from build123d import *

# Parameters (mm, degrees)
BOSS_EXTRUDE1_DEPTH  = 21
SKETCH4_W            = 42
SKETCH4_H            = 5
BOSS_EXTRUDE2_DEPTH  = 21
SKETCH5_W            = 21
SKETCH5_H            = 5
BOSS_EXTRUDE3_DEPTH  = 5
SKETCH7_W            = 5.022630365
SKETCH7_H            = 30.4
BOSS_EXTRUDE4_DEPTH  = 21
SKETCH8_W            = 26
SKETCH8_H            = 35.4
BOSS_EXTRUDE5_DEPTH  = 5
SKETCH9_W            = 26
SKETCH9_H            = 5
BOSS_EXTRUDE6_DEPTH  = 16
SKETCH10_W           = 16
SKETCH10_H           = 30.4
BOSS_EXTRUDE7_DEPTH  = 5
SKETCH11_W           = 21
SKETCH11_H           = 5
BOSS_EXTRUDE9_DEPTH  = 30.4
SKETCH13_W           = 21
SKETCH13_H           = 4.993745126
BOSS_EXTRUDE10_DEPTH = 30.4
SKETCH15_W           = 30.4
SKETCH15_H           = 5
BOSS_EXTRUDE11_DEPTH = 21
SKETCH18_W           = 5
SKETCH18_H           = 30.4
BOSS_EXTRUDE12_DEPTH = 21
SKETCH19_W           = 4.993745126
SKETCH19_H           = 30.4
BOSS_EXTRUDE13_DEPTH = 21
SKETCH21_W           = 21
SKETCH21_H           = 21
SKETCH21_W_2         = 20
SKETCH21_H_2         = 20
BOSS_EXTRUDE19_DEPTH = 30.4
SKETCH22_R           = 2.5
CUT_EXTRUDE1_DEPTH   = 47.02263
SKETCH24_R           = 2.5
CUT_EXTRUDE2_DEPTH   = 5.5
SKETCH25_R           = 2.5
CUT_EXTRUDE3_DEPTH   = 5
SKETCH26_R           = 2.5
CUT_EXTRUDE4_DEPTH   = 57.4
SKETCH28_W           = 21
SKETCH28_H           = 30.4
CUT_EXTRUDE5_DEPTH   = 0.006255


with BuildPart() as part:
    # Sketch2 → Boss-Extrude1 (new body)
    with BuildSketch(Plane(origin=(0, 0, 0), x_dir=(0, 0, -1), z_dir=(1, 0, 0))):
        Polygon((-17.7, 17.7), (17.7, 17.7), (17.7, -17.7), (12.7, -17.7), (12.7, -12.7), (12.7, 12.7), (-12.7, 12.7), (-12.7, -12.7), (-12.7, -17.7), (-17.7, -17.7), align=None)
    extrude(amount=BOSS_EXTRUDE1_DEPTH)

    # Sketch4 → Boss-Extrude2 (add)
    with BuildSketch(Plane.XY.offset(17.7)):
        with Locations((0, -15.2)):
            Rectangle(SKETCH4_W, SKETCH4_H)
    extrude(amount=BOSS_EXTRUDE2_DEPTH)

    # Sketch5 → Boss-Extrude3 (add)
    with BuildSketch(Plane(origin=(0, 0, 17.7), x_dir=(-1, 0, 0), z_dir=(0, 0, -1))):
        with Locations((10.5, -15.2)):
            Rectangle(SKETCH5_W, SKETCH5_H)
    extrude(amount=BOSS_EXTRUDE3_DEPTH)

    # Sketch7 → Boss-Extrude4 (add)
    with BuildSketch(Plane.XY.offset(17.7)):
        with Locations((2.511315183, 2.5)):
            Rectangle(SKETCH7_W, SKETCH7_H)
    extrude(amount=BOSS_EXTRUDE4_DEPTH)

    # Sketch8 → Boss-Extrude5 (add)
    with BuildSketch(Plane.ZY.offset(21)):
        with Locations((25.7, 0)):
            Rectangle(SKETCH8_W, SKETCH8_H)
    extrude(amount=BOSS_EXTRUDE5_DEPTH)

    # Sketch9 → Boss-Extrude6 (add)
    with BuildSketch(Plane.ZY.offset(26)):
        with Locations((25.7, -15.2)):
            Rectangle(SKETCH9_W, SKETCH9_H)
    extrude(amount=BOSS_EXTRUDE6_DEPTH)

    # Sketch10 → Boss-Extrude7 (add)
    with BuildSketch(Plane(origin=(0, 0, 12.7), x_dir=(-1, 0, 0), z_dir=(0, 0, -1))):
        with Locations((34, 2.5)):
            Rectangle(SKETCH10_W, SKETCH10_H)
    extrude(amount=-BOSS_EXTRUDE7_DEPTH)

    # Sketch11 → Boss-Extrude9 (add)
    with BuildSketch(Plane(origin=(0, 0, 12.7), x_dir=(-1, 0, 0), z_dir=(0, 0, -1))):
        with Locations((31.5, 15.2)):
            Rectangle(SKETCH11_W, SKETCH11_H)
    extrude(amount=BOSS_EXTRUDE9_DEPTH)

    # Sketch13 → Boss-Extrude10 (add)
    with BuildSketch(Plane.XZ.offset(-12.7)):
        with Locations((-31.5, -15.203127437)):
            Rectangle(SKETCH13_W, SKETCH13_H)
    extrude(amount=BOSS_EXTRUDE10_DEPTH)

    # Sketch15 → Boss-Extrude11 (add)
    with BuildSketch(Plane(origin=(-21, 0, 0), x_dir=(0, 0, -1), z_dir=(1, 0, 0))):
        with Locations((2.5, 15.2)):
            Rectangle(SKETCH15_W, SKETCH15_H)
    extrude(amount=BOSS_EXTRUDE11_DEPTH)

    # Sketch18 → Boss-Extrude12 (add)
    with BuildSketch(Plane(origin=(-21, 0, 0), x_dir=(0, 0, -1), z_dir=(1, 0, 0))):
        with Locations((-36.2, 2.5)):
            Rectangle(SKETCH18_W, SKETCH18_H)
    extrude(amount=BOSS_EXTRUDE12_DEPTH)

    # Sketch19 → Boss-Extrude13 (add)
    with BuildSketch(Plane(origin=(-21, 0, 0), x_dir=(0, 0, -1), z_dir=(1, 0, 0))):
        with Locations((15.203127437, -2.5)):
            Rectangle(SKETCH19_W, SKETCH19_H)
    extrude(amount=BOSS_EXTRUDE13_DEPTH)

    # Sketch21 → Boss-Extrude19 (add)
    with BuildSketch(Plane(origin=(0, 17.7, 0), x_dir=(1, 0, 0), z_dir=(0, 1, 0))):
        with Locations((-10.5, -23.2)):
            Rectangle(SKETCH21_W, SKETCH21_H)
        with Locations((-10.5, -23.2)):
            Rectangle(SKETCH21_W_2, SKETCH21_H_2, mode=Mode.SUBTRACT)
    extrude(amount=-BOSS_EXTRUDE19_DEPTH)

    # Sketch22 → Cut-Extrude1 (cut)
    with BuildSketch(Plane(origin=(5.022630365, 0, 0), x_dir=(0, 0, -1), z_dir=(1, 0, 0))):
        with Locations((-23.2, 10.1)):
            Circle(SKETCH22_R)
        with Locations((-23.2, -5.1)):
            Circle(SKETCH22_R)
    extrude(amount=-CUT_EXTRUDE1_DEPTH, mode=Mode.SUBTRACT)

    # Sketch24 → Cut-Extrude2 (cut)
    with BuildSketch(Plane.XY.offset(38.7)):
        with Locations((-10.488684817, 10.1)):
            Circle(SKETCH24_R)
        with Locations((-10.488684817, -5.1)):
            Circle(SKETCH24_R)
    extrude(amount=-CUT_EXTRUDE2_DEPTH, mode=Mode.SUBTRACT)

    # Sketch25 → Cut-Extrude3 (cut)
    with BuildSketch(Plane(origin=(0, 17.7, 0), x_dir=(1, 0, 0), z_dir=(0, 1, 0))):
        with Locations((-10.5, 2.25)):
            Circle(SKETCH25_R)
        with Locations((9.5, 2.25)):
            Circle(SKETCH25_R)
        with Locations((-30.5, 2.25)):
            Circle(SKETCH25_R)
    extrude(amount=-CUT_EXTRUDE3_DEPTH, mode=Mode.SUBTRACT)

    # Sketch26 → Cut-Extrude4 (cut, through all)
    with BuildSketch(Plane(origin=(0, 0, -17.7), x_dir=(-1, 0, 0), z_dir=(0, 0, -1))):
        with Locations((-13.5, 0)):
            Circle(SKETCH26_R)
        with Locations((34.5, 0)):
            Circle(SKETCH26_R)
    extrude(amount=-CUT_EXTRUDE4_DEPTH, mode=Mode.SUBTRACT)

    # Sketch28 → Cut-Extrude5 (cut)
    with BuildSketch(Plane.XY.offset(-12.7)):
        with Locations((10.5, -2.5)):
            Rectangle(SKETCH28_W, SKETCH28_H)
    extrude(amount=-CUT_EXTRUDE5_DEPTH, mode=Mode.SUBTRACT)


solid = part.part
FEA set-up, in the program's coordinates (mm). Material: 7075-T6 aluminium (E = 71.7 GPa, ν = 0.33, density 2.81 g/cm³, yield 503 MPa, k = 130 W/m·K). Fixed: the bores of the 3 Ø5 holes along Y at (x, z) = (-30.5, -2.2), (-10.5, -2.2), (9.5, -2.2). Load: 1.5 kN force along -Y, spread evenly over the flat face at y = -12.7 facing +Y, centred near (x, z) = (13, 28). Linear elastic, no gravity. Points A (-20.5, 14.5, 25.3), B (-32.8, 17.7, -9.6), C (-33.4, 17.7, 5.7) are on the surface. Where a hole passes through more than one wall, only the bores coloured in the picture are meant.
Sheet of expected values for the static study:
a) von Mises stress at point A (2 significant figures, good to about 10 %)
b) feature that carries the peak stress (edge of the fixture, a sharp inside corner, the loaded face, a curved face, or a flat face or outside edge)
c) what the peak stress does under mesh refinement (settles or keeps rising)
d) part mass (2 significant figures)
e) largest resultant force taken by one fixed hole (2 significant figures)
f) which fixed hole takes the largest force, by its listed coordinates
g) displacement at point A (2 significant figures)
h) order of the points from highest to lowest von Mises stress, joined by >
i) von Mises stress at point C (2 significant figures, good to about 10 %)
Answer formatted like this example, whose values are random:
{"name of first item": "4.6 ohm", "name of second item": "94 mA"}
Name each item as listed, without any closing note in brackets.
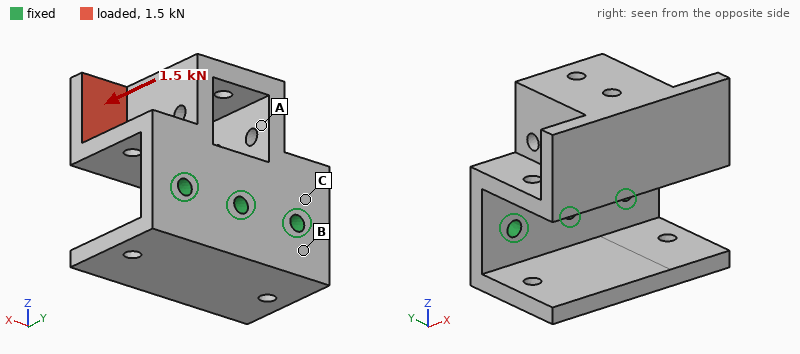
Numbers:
{"von Mises stress at point A": "33 MPa", "feature that carries the peak stress": "edge of the fixture", "what the peak stress does under mesh refinement": "keeps rising", "part mass": "120 g", "largest resultant force taken by one fixed hole": "1.2 kN", "which fixed hole takes the largest force, by its listed coordinates": "(9.5, -2.2)", "displacement at point A": "0.24 mm", "order of the points from highest to lowest von Mises stress, joined by >": "C > A > B", "von Mises stress at point C": "100 MPa"}
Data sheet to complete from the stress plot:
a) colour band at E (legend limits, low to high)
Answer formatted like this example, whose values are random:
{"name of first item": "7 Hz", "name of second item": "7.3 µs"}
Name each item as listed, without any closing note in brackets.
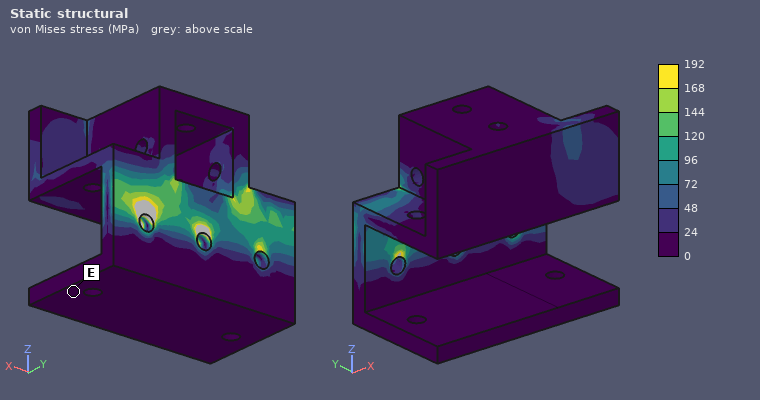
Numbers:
{"colour band at E": "0 to 24 MPa"}
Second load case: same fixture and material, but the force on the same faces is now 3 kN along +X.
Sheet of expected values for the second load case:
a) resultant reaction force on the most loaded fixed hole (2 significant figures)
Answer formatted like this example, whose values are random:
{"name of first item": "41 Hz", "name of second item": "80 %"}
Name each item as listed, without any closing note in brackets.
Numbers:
{"resultant reaction force on the most loaded fixed hole": "3.0 kN"}
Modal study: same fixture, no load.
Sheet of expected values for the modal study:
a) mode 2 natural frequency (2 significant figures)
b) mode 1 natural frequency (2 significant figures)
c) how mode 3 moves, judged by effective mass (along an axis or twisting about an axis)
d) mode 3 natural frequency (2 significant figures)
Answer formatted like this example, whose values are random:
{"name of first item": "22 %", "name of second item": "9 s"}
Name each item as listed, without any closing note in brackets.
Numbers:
{"mode 2 natural frequency": "2500 Hz", "mode 1 natural frequency": "970 Hz", "how mode 3 moves, judged by effective mass": "along X", "mode 3 natural frequency": "3000 Hz"}
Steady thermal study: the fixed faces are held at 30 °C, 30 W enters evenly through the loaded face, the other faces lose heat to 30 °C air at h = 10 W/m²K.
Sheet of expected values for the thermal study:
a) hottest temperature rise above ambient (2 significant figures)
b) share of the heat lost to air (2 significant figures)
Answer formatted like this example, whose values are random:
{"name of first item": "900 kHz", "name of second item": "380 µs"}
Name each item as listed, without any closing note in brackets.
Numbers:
{"hottest temperature rise above ambient": "54 K", "share of the heat lost to air": "10 %"}
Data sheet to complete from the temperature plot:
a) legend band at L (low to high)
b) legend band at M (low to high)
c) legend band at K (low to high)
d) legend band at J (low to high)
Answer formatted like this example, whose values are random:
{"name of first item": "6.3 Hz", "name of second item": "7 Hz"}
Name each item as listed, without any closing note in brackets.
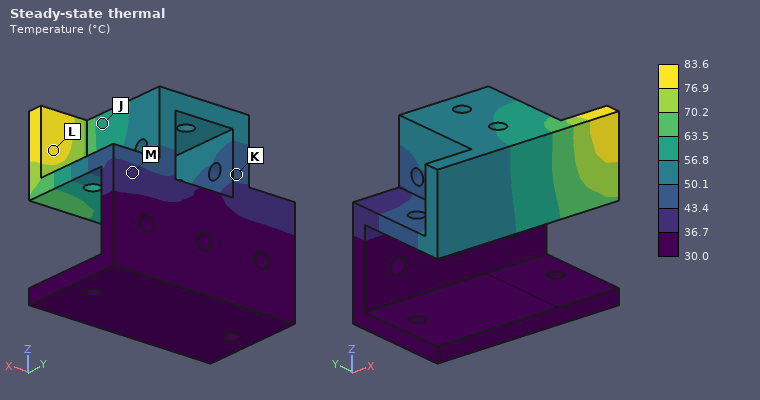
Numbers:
{"legend band at L": "76.9 to 83.6 °C", "legend band at M": "36.7 to 43.4 °C", "legend band at K": "43.4 to 50.1 °C", "legend band at J": "56.8 to 63.5 °C"}
